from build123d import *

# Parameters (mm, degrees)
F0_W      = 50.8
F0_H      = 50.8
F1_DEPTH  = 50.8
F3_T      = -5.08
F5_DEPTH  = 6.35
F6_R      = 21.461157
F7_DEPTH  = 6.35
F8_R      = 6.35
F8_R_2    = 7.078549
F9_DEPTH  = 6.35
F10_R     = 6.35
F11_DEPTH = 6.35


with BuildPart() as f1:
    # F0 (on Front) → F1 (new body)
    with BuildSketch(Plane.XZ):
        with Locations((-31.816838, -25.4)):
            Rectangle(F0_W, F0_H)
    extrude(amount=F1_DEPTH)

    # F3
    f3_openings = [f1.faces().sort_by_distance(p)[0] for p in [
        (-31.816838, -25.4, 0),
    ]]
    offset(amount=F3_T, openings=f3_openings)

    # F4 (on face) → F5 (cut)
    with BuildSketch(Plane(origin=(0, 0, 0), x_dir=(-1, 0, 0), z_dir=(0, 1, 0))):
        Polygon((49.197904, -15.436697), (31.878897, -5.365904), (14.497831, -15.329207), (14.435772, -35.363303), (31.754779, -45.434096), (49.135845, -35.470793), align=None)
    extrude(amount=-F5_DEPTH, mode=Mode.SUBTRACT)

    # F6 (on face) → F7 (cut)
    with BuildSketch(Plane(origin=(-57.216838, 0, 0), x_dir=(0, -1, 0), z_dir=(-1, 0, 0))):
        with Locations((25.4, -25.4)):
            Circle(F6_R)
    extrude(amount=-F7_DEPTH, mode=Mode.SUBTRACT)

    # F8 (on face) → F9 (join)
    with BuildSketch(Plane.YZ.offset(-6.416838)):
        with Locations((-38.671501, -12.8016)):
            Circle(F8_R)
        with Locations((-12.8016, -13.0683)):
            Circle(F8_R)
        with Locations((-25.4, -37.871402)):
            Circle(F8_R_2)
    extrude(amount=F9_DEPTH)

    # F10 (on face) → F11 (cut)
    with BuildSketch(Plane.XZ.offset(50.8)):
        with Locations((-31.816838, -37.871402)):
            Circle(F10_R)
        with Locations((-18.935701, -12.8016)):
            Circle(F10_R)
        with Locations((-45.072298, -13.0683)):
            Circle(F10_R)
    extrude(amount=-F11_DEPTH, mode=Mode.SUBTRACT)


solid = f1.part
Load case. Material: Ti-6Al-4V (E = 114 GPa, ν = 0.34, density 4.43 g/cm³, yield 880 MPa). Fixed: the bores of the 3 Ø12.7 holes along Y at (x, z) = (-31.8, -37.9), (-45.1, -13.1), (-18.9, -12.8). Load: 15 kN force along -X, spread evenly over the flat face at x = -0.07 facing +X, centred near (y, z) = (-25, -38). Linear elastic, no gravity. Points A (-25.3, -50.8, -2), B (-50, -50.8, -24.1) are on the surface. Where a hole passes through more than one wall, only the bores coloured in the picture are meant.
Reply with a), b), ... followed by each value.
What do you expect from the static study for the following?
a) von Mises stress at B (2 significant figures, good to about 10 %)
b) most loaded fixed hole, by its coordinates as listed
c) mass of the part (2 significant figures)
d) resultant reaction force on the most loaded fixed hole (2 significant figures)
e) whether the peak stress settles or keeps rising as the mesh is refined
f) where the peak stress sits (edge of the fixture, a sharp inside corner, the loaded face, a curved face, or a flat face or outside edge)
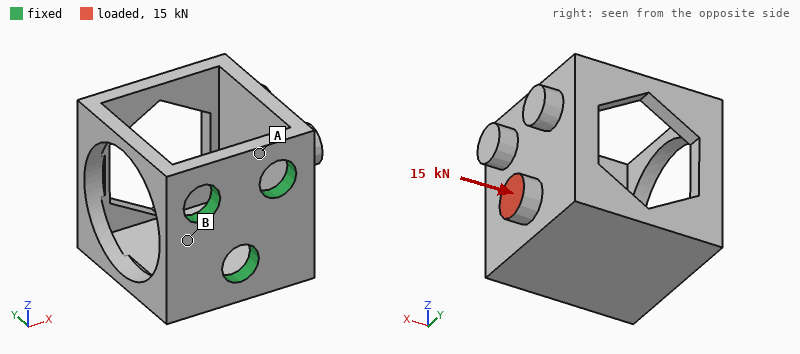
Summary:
a) 190 MPa
b) (-31.8, -37.9)
c) 190 g
d) 12 kN
e) keeps rising
f) edge of the fixture
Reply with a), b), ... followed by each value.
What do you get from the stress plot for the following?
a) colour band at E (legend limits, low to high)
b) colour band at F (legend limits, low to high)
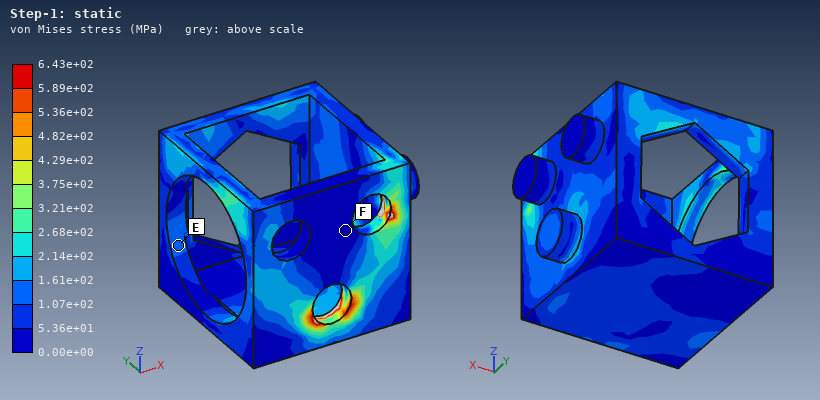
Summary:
a) 1.07e+02 to 1.61e+02 MPa
b) 0.00e+00 to 5.36e+01 MPa
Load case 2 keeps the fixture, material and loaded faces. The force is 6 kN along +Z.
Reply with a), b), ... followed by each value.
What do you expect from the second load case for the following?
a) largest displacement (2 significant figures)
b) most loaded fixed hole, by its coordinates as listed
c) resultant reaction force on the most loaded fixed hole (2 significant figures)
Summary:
a) 0.17 mm
b) (-18.9, -12.8)
c) 6.9 kN
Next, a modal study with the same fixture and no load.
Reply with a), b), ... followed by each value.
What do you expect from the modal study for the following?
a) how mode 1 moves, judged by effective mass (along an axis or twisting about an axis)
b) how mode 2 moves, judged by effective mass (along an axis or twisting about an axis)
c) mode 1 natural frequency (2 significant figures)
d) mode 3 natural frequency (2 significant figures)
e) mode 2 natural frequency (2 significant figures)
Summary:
a) along X
b) along Z
c) 1900 Hz
d) 6000 Hz
e) 2700 Hz
